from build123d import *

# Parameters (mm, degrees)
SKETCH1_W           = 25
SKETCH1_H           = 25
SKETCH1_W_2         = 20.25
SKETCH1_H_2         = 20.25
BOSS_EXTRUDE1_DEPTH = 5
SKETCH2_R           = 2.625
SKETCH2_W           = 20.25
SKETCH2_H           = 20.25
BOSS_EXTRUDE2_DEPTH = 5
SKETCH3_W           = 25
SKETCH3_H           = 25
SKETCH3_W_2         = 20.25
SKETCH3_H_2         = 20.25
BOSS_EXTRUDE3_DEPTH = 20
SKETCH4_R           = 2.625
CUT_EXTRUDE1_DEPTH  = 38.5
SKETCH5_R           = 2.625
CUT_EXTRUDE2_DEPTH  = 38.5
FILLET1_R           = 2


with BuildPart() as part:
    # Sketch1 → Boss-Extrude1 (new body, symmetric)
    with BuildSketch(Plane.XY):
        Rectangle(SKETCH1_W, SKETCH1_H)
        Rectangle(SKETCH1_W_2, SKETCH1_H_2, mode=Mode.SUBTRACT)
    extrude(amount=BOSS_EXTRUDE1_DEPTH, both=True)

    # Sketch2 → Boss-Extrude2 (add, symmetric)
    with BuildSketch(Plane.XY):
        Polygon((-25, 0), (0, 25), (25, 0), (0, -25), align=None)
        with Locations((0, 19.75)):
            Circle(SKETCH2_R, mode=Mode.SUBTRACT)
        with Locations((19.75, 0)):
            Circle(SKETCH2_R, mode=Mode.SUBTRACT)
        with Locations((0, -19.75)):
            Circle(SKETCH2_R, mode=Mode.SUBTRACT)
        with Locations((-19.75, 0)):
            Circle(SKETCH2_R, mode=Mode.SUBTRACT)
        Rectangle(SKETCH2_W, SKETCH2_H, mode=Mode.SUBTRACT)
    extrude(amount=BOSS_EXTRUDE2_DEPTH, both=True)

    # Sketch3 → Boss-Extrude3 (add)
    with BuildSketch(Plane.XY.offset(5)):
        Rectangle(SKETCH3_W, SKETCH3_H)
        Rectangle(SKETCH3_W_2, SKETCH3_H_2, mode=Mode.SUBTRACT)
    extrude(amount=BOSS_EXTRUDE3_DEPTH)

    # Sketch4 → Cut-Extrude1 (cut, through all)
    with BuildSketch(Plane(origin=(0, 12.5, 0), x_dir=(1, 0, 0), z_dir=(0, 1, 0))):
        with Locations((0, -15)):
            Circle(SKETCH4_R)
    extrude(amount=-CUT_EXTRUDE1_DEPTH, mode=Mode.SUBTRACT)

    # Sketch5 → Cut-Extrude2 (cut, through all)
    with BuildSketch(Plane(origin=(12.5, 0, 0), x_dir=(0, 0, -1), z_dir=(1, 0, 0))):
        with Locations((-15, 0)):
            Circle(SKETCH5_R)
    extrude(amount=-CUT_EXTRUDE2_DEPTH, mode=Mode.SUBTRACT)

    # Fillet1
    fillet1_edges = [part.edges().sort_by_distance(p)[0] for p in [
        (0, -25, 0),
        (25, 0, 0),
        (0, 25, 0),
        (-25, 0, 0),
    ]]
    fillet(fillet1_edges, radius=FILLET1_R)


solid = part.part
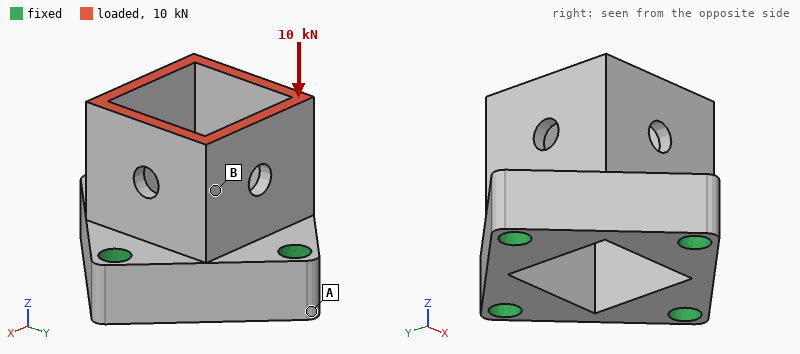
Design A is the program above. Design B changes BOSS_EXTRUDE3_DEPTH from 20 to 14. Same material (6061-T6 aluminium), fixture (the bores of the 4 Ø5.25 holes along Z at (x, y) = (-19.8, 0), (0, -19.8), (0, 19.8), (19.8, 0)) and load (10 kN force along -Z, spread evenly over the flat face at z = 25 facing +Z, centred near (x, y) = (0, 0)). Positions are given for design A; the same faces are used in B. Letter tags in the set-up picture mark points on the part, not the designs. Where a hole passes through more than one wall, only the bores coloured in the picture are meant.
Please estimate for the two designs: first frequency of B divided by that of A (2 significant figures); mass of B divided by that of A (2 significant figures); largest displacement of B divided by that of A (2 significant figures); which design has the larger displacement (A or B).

1.3
0.89
1.2
B
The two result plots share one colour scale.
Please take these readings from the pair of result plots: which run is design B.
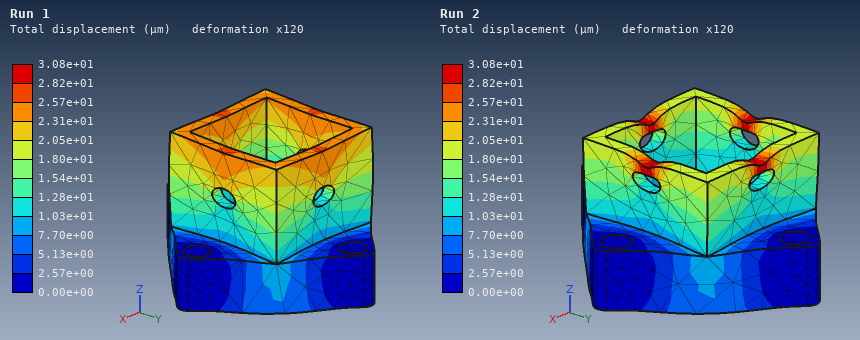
Run 2
